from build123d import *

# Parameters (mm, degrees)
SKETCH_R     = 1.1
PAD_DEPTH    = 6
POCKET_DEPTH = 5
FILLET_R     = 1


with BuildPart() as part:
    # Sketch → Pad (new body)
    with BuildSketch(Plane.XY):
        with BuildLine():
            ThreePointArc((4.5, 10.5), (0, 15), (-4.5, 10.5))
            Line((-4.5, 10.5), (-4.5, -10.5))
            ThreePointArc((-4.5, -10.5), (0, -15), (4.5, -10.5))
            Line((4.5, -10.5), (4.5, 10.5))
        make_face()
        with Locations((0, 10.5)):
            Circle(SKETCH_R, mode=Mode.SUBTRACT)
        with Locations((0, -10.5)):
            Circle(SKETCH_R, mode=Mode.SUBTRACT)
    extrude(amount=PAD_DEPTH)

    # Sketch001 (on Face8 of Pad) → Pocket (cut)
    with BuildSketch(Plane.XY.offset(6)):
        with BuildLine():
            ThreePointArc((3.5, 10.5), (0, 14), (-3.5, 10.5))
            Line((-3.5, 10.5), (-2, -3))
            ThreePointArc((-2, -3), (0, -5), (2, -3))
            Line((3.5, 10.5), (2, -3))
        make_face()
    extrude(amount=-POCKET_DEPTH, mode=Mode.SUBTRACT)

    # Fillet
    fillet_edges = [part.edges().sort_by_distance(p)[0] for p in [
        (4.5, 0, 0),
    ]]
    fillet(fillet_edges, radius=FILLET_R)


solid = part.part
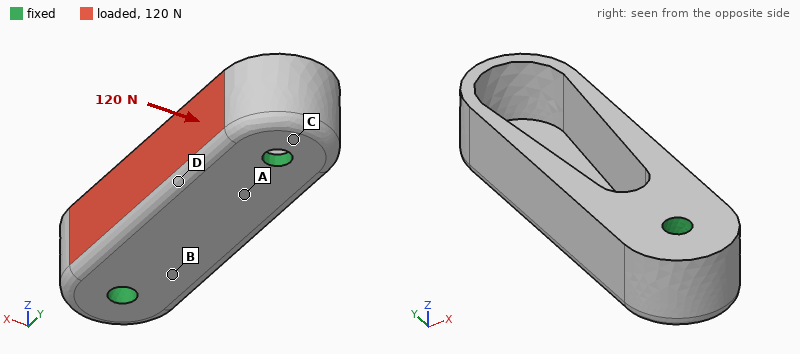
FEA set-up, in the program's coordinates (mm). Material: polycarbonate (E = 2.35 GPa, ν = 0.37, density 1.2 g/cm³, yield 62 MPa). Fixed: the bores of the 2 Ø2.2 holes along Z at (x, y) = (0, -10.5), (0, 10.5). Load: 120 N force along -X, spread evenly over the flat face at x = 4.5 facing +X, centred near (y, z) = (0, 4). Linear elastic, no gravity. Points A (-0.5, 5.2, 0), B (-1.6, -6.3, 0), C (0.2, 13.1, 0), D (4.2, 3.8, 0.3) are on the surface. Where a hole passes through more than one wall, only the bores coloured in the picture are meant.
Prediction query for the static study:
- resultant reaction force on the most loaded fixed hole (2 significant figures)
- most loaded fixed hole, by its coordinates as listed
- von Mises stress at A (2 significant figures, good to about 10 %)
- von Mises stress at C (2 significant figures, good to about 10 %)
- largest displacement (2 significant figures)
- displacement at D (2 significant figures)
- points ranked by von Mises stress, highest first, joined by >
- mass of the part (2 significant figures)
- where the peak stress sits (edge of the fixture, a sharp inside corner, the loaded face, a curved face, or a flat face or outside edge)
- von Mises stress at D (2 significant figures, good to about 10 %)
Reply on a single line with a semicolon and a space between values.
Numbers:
71 N; (0, -10.5); 6.7 MPa; 4.5 MPa; 0.33 mm; 0.073 mm; D > A > C > B; 1.2 g; a flat face or outside edge; 10 MPa
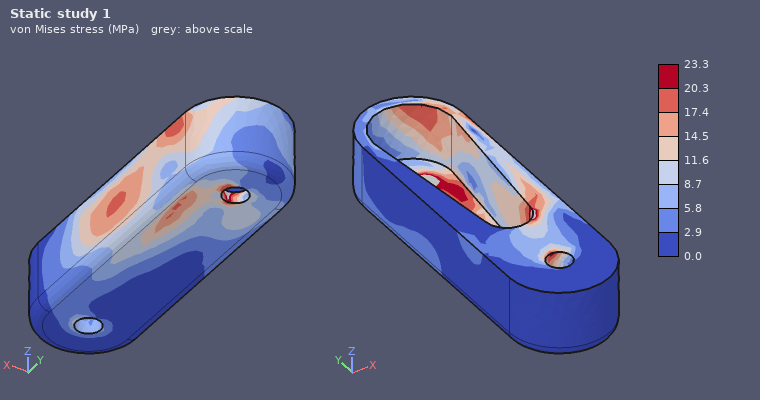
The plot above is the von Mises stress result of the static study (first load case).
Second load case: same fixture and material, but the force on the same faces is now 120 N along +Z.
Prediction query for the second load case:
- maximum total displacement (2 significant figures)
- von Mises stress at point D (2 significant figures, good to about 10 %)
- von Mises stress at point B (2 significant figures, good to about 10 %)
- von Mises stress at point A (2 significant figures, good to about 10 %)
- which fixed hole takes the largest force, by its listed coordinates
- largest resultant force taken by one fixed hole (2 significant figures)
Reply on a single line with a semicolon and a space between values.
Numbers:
0.32 mm; 9.7 MPa; 6.3 MPa; 6.9 MPa; (0, -10.5); 83 N
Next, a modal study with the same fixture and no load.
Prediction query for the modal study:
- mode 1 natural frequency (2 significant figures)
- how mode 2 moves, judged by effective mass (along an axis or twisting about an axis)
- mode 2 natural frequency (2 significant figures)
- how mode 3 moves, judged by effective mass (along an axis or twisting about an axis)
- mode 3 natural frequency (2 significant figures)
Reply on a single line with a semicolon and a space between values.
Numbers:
6100 Hz; along Z; 8100 Hz; along X; 9600 Hz
